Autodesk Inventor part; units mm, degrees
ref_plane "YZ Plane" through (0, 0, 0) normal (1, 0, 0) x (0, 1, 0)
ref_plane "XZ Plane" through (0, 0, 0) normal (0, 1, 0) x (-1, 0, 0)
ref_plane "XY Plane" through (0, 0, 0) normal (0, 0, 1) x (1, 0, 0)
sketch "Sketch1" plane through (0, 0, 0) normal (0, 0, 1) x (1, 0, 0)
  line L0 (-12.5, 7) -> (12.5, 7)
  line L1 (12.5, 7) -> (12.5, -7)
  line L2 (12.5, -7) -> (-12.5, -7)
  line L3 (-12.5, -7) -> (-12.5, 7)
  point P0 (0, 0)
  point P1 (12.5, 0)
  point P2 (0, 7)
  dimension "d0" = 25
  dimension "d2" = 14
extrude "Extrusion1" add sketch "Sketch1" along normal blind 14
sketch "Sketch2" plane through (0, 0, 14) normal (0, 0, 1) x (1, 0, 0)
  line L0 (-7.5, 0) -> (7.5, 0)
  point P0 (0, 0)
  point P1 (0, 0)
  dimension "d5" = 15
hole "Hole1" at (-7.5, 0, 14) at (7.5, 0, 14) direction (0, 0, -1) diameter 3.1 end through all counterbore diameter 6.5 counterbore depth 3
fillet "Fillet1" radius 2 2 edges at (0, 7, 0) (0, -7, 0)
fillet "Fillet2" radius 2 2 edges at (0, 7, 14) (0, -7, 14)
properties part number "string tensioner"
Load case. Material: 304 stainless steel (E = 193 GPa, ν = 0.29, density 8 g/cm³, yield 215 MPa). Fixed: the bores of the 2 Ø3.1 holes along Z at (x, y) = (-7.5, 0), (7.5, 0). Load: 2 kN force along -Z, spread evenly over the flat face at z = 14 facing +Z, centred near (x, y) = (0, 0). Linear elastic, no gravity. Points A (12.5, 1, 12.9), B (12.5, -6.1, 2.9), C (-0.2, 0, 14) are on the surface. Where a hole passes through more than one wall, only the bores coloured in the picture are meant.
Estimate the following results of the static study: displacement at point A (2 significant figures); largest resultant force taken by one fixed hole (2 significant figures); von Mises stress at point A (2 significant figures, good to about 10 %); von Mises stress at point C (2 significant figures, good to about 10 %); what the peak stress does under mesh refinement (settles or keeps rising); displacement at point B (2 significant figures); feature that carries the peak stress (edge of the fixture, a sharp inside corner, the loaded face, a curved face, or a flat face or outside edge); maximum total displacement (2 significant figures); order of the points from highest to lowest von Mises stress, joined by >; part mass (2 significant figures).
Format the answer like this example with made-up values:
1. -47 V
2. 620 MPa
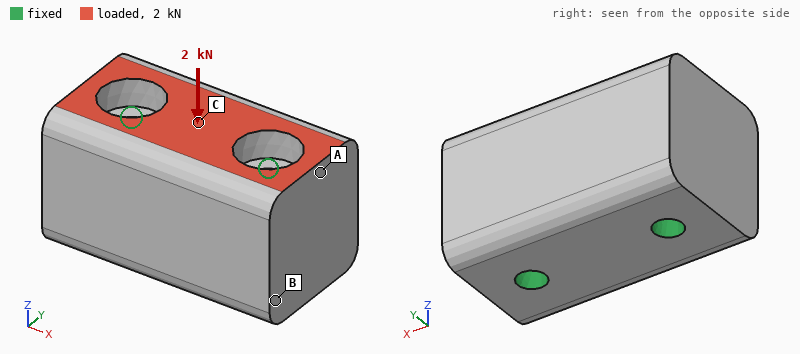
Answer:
1. 0.49 µm
2. 1.0 kN
3. 11 MPa
4. 6.9 MPa
5. keeps rising
6. 0.23 µm
7. edge of the fixture
8. 0.63 µm
9. A > C > B
10. 36 g
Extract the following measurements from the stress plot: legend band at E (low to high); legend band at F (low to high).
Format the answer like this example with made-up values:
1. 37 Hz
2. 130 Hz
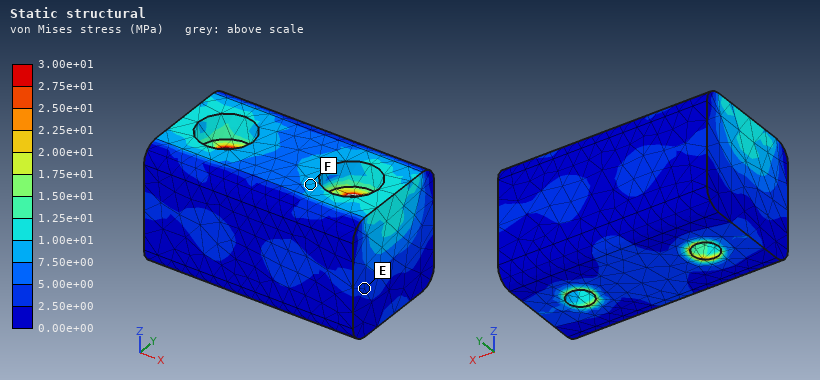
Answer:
1. 2.50e+00 to 5.00e+00 MPa
2. 7.50e+00 to 1.00e+01 MPa
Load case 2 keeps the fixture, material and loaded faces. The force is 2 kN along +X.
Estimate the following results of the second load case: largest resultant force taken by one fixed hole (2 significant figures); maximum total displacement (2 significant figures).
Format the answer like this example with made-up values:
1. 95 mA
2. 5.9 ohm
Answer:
1. 1.2 kN
2. 2.2 µm
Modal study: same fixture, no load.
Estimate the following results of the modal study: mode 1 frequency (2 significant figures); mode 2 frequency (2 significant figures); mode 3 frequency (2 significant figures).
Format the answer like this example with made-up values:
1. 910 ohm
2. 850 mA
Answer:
1. 56 kHz
2. 71 kHz
3. 73 kHz
